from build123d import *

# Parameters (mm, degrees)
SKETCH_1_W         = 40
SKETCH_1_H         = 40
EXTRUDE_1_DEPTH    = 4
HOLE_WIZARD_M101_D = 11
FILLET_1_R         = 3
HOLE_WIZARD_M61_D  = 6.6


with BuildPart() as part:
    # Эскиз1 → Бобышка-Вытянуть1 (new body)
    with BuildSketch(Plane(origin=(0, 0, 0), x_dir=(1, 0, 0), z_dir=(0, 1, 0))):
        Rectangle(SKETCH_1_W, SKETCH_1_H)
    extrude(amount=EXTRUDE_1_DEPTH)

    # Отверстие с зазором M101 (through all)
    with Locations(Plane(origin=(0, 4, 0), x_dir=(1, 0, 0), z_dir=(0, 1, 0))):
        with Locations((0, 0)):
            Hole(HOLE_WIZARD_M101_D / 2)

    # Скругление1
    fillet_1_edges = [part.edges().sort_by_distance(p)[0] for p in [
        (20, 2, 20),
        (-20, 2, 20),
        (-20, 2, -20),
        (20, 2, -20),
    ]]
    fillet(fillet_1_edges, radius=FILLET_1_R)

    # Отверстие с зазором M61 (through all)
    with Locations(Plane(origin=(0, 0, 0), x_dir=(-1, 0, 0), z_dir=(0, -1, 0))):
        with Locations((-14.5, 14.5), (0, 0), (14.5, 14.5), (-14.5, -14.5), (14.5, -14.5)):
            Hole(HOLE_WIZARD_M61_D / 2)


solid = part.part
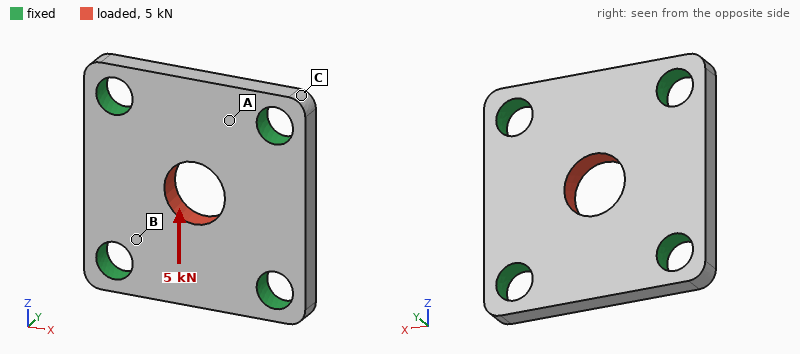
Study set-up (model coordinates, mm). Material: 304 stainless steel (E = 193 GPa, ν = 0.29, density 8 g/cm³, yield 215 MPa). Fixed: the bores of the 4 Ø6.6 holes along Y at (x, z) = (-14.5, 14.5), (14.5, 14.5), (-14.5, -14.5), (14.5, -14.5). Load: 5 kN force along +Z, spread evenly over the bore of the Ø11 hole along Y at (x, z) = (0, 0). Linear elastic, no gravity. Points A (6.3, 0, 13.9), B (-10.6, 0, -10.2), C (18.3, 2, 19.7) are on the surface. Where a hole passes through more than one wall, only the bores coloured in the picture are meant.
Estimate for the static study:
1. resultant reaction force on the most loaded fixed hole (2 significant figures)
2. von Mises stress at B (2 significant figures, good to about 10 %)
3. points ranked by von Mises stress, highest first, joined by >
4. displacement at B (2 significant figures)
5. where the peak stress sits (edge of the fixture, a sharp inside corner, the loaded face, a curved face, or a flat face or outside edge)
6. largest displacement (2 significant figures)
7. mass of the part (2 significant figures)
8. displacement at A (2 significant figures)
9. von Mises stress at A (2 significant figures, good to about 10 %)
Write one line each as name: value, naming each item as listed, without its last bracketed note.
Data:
resultant reaction force on the most loaded fixed hole: 1.4 kN
von Mises stress at B: 36 MPa
points ranked by von Mises stress, highest first, joined by >: B > A > C
displacement at B: 0.62 µm
where the peak stress sits: edge of the fixture
largest displacement: 3.1 µm
mass of the part: 44 g
displacement at A: 1.4 µm
von Mises stress at A: 24 MPa
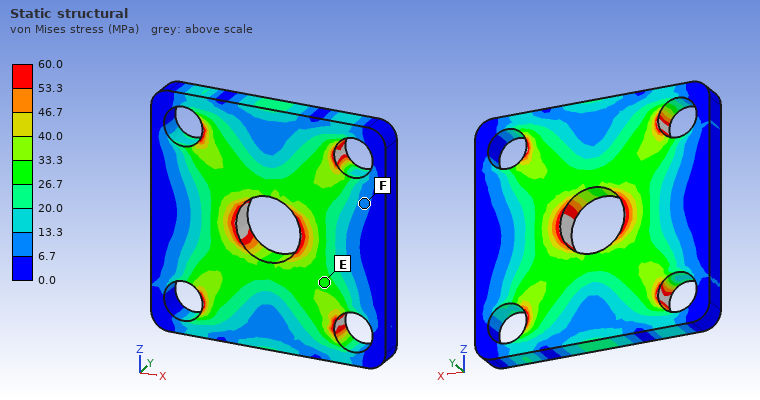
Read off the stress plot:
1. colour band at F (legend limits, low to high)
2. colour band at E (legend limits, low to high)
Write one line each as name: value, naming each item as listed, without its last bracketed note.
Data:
colour band at F: 6.7 to 13.3 MPa
colour band at E: 26.7 to 33.3 MPa
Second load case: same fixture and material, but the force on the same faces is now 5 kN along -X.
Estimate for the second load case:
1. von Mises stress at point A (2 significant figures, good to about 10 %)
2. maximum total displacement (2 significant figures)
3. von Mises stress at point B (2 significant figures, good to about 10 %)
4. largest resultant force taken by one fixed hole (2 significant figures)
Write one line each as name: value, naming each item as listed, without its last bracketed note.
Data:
von Mises stress at point A: 17 MPa
maximum total displacement: 3.1 µm
von Mises stress at point B: 37 MPa
largest resultant force taken by one fixed hole: 1.4 kN
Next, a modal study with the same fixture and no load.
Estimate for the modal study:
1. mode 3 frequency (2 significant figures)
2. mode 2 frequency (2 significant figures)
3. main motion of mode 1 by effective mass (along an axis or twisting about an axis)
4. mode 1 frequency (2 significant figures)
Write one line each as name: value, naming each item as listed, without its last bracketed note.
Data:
mode 3 frequency: 30 kHz
mode 2 frequency: 30 kHz
main motion of mode 1 by effective mass: along Y
mode 1 frequency: 22 kHz
